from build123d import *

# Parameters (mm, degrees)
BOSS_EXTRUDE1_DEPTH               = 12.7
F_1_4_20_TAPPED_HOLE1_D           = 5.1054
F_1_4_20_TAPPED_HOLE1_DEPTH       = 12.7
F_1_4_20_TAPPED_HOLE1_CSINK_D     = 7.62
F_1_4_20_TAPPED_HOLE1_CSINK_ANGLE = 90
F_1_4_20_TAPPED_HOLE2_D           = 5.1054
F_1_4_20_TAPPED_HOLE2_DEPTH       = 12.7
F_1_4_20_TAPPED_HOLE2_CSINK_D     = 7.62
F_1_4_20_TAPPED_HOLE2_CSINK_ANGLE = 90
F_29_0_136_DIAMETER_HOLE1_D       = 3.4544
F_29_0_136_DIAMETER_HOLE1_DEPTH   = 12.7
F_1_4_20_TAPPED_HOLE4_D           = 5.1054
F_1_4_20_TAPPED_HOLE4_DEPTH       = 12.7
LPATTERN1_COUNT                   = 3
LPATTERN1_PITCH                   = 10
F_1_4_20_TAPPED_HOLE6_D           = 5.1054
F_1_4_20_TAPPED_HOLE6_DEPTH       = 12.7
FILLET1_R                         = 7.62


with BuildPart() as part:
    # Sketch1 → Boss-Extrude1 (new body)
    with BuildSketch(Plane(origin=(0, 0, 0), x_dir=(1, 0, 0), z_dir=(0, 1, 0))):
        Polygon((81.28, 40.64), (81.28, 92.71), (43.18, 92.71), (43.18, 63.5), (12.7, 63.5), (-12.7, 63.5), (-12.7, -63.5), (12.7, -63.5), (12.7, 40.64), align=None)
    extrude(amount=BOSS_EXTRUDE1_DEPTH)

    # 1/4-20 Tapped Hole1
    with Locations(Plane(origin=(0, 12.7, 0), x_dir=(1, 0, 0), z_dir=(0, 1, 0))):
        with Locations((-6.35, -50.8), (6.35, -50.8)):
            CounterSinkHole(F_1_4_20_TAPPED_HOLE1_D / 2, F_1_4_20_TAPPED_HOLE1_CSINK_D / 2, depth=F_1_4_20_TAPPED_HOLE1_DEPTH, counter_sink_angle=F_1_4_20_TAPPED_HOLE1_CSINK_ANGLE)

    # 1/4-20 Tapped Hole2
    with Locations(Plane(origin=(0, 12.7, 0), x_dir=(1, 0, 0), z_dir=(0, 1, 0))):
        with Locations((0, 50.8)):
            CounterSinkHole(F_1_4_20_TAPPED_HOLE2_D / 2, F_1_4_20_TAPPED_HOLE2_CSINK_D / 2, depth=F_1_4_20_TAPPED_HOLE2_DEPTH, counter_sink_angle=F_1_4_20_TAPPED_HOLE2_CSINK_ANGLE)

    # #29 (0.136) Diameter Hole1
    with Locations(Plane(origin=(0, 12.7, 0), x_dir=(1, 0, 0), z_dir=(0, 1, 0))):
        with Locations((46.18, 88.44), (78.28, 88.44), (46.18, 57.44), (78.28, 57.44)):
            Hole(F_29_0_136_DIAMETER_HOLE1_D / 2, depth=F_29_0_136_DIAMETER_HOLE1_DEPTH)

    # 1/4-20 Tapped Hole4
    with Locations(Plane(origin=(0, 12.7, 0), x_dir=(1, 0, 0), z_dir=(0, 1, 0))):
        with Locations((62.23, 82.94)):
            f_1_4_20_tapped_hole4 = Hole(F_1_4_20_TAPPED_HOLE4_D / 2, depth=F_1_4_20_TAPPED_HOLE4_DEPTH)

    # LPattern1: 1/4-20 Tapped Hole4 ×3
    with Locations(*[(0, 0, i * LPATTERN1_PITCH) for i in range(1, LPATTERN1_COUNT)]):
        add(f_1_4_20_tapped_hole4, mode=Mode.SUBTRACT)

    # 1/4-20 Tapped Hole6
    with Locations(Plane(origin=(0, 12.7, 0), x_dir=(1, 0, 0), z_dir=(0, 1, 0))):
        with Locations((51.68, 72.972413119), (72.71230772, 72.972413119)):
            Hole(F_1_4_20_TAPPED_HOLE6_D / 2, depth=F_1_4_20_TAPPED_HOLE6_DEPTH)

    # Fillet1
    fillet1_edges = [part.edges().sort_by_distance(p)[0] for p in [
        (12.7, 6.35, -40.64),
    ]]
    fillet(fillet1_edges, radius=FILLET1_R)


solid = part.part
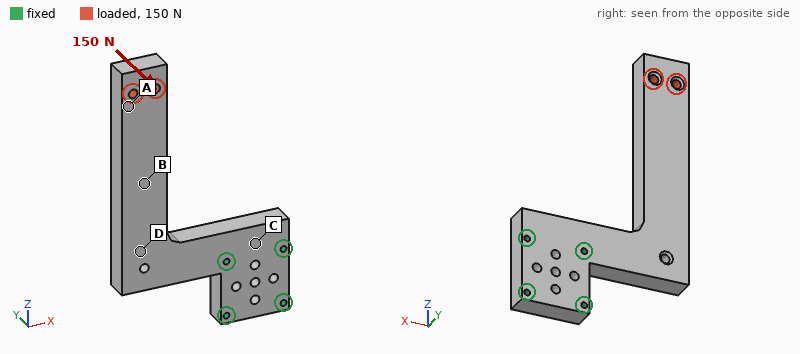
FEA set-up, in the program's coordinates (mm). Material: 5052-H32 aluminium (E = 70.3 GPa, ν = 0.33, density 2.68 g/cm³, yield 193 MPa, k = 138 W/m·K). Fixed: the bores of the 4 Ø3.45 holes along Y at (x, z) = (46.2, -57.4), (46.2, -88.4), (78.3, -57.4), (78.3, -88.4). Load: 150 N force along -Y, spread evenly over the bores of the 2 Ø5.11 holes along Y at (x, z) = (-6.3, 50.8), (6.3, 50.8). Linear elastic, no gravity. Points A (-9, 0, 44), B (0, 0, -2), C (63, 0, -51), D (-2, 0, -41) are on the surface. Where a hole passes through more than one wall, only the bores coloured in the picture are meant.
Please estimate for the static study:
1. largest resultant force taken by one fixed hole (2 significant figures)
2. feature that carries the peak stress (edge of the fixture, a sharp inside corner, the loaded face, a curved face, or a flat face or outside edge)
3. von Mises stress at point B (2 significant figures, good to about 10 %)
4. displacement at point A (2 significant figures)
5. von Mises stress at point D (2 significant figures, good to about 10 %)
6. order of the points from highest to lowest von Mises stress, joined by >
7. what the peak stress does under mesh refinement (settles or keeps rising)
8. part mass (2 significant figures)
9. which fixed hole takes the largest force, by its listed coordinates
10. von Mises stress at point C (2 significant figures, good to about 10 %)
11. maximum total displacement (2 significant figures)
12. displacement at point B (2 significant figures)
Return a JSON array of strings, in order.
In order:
["360 N", "edge of the fixture", "12 MPa", "0.41 mm", "15 MPa", "D > B > C > A", "keeps rising", "190 g", "(46.2, -57.4)", "5.7 MPa", "0.50 mm", "0.19 mm"]
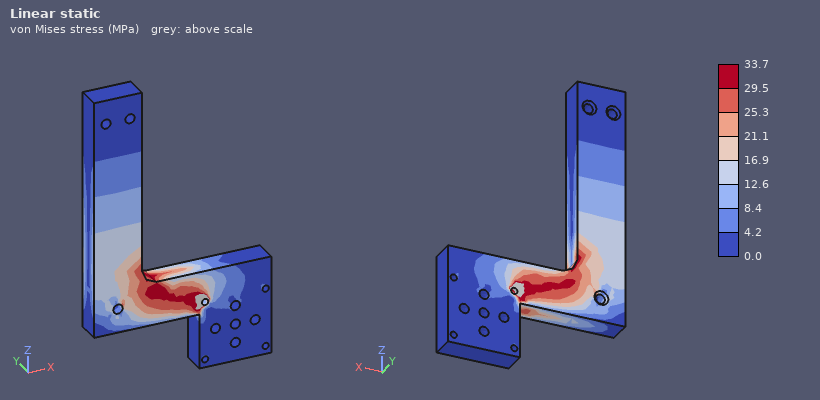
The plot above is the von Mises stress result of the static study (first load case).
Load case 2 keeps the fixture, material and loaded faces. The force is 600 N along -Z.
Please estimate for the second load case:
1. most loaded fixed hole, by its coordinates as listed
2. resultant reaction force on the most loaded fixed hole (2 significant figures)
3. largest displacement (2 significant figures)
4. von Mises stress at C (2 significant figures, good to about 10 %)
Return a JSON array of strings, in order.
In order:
["(46.2, -57.4)", "1.3 kN", "0.13 mm", "6.9 MPa"]
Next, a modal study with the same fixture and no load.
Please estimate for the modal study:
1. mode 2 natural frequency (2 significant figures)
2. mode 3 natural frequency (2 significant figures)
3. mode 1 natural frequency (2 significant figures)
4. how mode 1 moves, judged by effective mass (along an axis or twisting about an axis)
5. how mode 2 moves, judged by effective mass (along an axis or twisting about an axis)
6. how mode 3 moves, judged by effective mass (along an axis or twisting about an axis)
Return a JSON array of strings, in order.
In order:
["830 Hz", "1900 Hz", "480 Hz", "along Y", "along X", "along Y"]
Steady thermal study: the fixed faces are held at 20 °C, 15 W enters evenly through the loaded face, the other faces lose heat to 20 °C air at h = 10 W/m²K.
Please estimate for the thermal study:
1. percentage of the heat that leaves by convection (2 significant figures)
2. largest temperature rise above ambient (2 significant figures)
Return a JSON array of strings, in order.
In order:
["19 %", "43 K"]
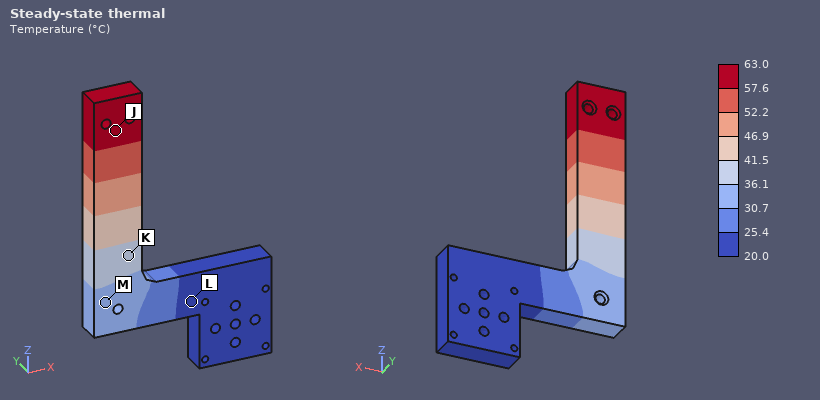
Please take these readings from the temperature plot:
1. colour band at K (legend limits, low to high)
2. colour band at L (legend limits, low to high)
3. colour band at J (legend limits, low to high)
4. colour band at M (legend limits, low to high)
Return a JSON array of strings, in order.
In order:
["36.1 to 41.5 °C", "20.0 to 25.4 °C", "57.6 to 63.0 °C", "30.7 to 36.1 °C"]
